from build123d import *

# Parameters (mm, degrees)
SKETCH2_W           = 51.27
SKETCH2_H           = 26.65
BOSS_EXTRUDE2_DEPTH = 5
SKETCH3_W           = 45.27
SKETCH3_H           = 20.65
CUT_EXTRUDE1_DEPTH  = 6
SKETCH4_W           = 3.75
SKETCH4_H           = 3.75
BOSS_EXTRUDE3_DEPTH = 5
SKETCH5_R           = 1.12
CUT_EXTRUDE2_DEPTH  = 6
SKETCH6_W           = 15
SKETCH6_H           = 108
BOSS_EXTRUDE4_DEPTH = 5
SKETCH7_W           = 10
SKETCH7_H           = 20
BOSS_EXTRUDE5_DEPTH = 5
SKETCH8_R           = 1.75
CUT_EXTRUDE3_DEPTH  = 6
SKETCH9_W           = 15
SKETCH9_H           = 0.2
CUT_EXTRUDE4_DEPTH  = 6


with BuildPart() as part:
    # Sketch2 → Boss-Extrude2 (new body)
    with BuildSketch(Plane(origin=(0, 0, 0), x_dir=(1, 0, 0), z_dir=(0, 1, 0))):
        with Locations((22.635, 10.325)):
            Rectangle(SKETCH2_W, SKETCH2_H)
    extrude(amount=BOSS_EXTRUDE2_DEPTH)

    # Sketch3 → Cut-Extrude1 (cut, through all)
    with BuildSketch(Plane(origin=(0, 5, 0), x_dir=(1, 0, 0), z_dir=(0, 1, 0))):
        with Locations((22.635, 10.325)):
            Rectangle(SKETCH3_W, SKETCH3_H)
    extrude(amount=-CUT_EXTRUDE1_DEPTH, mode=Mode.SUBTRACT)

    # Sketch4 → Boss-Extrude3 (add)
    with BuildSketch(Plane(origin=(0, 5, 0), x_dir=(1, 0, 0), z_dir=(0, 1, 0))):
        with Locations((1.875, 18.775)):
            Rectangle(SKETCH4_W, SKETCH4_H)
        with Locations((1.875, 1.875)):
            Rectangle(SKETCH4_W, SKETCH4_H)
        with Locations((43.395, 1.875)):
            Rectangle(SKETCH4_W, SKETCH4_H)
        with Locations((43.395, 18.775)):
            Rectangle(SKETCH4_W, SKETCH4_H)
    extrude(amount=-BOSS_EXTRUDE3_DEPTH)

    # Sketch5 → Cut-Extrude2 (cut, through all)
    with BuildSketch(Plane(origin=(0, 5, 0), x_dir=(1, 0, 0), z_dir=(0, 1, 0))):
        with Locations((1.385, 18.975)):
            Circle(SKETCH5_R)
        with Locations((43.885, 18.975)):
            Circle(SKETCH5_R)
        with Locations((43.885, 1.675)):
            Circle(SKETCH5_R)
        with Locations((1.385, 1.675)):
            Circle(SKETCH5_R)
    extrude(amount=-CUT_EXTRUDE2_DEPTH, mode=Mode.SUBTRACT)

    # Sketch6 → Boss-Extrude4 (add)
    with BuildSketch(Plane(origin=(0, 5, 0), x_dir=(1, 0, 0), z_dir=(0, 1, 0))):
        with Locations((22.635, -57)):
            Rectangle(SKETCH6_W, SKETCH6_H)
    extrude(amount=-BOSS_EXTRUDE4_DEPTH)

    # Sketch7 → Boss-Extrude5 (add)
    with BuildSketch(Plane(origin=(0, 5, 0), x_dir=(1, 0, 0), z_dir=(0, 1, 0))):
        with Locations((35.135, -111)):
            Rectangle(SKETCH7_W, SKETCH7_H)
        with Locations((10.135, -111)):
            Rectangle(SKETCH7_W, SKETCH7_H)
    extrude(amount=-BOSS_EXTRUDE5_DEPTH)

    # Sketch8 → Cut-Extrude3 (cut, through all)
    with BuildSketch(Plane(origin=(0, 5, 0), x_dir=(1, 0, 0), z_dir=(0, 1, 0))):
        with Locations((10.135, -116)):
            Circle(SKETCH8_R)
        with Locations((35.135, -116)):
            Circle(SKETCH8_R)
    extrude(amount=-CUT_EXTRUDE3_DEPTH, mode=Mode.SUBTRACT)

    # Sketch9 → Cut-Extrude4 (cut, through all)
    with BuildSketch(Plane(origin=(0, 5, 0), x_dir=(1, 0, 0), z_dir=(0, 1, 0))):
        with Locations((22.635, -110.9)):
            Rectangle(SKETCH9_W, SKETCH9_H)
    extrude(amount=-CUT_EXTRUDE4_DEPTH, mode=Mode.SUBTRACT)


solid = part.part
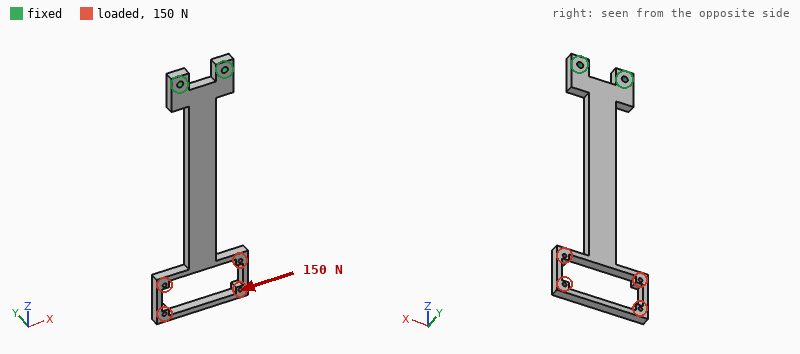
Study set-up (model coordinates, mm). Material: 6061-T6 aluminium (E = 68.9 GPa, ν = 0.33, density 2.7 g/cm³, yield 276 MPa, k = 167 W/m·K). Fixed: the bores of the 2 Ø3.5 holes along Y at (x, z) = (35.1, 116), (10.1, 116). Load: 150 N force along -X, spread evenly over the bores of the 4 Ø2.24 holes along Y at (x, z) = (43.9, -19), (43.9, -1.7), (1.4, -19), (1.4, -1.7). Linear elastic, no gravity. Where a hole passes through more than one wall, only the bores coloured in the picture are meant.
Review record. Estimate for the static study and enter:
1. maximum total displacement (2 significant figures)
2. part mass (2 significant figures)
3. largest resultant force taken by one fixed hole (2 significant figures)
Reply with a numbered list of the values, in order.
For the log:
1. 1.3 mm
2. 33 g
3. 800 N
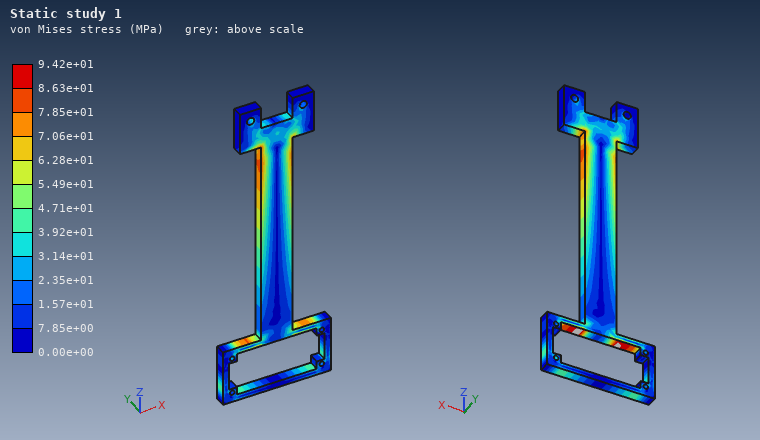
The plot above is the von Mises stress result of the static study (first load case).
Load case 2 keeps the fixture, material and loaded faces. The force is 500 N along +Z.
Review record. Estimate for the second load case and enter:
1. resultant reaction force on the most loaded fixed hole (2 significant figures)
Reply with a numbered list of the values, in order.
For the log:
1. 270 N
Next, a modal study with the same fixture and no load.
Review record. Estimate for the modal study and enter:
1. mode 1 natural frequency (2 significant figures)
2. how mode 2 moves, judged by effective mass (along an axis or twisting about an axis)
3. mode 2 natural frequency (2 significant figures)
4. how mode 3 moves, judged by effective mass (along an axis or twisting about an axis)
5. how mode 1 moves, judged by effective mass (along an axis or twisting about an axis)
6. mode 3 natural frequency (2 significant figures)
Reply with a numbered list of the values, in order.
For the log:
1. 200 Hz
2. along X
3. 630 Hz
4. twisting about Z
5. along Y
6. 1100 Hz
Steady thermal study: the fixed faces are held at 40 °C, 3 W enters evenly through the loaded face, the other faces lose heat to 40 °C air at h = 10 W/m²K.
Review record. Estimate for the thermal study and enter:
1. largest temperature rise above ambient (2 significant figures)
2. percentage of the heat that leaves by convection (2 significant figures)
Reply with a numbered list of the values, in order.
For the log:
1. 31 K
2. 35 %
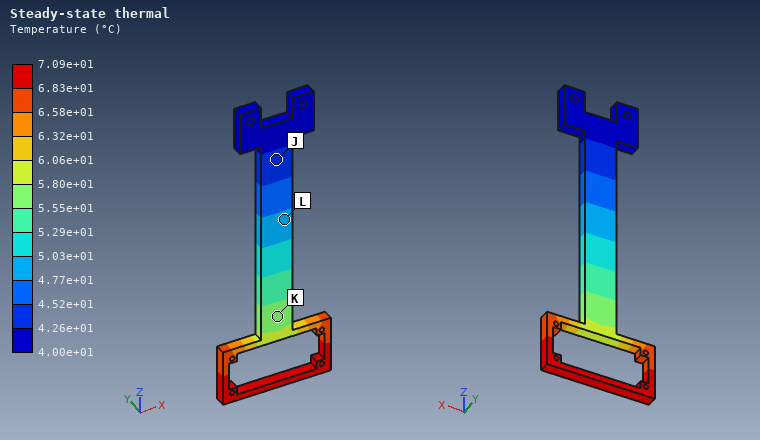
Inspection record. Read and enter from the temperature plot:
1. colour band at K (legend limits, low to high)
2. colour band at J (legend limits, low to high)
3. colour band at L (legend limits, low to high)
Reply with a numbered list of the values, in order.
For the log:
1. 5.55e+01 to 5.80e+01 °C
2. 4.26e+01 to 4.52e+01 °C
3. 4.77e+01 to 5.03e+01 °C
